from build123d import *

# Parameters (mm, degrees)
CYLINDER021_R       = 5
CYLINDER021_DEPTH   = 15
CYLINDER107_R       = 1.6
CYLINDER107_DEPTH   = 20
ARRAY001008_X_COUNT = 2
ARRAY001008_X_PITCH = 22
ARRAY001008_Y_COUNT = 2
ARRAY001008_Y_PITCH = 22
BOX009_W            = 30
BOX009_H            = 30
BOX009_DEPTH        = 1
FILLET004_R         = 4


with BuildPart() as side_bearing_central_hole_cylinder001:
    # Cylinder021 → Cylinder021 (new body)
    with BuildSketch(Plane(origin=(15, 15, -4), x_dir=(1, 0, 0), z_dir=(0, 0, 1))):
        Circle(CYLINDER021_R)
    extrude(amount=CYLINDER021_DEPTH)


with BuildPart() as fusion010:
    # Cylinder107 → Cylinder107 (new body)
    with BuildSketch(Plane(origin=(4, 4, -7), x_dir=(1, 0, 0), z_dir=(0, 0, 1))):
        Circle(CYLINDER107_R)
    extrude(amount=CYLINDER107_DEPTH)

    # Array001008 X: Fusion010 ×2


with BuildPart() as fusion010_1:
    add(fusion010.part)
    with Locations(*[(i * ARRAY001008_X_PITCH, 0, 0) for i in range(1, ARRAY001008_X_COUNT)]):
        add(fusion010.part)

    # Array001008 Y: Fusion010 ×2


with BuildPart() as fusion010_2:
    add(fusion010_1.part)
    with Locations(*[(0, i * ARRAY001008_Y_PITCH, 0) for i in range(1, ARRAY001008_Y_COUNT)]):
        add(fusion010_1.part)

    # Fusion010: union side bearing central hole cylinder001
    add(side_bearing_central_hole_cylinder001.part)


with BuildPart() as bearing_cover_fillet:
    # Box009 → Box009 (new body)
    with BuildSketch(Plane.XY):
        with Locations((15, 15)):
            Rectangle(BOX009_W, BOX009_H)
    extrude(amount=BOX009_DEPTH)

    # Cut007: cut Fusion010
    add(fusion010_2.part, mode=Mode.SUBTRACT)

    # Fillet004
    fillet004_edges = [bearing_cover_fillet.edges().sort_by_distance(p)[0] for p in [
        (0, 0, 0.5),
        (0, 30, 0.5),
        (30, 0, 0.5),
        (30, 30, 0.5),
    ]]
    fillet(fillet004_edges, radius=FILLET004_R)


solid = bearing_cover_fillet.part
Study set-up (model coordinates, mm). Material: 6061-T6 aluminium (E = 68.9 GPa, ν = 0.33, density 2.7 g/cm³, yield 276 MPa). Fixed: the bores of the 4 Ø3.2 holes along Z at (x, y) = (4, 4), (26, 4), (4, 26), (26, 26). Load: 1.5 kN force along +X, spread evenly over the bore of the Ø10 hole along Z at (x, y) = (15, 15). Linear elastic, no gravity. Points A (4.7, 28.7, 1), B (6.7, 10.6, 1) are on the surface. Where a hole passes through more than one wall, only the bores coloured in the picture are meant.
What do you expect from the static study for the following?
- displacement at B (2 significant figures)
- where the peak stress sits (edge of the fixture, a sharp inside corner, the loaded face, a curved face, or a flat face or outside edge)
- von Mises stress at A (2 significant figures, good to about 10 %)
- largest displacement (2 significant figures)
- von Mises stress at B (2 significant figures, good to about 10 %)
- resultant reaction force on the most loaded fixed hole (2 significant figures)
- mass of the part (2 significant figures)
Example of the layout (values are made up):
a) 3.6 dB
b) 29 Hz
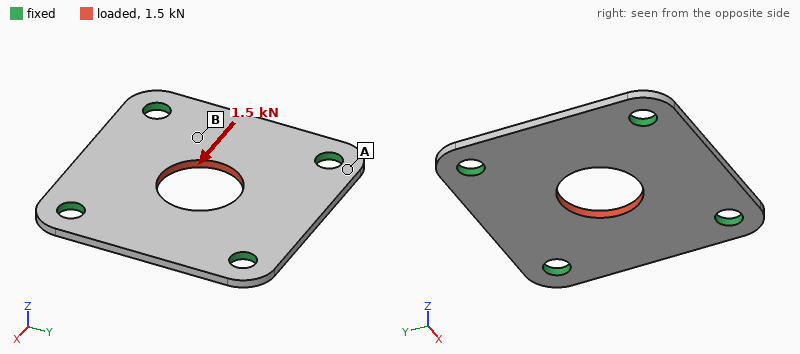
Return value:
a) 7.5 µm
b) edge of the fixture
c) 16 MPa
d) 12 µm
e) 44 MPa
f) 410 N
g) 2.1 g
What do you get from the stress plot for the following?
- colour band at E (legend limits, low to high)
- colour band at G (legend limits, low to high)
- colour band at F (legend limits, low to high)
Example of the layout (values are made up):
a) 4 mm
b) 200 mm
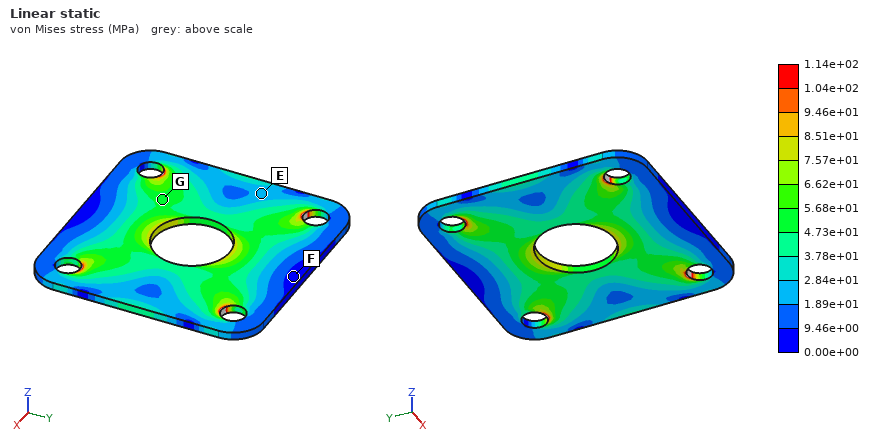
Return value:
a) 1.89e+01 to 2.84e+01 MPa
b) 4.73e+01 to 5.68e+01 MPa
c) 0.00e+00 to 9.46e+00 MPa
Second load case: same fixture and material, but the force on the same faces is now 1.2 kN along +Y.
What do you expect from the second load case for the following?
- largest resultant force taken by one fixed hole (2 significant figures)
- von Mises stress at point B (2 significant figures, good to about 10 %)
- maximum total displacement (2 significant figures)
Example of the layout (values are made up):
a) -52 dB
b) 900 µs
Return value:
a) 330 N
b) 35 MPa
c) 9.5 µm
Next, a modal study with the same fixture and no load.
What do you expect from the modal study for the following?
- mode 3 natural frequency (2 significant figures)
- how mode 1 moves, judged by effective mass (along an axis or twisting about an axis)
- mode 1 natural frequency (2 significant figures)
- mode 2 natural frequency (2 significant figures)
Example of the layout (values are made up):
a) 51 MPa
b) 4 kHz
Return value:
a) 14 kHz
b) along Z
c) 10 kHz
d) 14 kHz
